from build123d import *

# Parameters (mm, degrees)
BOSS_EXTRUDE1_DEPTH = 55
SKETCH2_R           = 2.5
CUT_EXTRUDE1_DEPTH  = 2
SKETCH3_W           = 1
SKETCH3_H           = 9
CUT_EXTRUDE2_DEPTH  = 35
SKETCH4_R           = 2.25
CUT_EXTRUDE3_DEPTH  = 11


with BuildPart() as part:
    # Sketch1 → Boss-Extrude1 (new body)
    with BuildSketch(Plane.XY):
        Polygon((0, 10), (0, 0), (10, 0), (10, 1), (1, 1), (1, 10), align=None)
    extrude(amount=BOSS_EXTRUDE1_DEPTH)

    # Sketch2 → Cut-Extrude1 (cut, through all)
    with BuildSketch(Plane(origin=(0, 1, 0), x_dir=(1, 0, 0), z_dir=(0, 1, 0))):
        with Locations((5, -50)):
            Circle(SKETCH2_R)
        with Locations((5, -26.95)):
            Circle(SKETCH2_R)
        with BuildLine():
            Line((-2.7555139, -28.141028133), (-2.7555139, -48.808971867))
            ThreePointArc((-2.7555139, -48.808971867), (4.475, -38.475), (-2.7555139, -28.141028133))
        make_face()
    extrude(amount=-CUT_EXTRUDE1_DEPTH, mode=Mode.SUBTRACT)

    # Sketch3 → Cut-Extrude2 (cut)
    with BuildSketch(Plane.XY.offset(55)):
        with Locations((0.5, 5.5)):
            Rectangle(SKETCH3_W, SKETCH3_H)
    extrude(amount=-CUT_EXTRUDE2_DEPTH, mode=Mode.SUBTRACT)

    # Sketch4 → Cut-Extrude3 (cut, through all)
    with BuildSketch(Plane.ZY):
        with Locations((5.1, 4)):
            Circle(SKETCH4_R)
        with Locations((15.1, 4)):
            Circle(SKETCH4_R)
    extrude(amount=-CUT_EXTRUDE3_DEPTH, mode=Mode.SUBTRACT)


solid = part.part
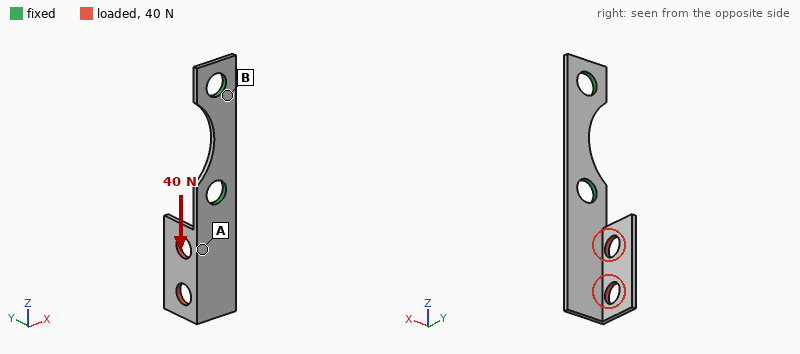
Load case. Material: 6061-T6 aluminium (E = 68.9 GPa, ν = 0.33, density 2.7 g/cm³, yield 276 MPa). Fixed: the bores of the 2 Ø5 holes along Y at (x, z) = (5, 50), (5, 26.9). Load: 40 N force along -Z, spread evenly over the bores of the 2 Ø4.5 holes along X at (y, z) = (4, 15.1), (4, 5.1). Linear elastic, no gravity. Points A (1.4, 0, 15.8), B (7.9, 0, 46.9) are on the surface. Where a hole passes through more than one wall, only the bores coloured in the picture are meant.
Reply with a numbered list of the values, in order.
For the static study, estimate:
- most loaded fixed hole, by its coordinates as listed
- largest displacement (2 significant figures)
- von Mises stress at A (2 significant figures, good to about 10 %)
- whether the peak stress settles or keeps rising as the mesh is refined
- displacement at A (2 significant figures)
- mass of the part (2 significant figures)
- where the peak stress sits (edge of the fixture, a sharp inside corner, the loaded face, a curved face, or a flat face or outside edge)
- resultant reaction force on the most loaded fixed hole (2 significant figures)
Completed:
1. (5, 26.9)
2. 0.44 mm
3. 19 MPa
4. keeps rising
5. 0.10 mm
6. 1.6 g
7. a sharp inside corner
8. 41 N
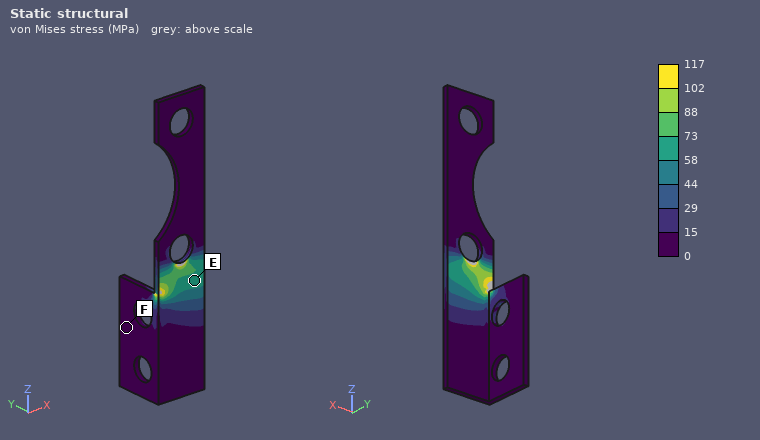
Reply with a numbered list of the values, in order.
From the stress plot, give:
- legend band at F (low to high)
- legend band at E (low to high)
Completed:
1. 0 to 15 MPa
2. 58 to 73 MPa
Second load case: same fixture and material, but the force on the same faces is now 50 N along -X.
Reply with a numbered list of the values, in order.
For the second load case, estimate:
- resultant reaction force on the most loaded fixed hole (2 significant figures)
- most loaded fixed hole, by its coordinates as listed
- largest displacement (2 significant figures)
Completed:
1. 54 N
2. (5, 26.9)
3. 0.34 mm
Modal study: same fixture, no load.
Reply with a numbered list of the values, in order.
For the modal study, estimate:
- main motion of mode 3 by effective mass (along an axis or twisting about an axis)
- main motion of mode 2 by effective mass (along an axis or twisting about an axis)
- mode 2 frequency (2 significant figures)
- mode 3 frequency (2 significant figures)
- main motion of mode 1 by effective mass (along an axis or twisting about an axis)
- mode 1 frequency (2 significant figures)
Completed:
1. along X
2. along X
3. 2900 Hz
4. 7900 Hz
5. along Y
6. 1100 Hz
